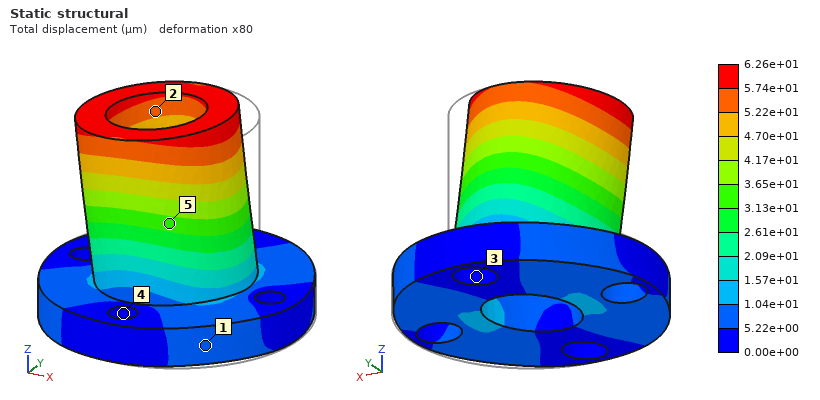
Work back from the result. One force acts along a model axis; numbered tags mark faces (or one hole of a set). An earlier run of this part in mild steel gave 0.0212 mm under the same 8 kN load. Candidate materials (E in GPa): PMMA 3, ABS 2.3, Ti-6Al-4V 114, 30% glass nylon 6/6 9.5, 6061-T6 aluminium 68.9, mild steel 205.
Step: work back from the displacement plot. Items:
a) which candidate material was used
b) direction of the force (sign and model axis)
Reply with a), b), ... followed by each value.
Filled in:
a) 6061-T6 aluminium
b) -X
